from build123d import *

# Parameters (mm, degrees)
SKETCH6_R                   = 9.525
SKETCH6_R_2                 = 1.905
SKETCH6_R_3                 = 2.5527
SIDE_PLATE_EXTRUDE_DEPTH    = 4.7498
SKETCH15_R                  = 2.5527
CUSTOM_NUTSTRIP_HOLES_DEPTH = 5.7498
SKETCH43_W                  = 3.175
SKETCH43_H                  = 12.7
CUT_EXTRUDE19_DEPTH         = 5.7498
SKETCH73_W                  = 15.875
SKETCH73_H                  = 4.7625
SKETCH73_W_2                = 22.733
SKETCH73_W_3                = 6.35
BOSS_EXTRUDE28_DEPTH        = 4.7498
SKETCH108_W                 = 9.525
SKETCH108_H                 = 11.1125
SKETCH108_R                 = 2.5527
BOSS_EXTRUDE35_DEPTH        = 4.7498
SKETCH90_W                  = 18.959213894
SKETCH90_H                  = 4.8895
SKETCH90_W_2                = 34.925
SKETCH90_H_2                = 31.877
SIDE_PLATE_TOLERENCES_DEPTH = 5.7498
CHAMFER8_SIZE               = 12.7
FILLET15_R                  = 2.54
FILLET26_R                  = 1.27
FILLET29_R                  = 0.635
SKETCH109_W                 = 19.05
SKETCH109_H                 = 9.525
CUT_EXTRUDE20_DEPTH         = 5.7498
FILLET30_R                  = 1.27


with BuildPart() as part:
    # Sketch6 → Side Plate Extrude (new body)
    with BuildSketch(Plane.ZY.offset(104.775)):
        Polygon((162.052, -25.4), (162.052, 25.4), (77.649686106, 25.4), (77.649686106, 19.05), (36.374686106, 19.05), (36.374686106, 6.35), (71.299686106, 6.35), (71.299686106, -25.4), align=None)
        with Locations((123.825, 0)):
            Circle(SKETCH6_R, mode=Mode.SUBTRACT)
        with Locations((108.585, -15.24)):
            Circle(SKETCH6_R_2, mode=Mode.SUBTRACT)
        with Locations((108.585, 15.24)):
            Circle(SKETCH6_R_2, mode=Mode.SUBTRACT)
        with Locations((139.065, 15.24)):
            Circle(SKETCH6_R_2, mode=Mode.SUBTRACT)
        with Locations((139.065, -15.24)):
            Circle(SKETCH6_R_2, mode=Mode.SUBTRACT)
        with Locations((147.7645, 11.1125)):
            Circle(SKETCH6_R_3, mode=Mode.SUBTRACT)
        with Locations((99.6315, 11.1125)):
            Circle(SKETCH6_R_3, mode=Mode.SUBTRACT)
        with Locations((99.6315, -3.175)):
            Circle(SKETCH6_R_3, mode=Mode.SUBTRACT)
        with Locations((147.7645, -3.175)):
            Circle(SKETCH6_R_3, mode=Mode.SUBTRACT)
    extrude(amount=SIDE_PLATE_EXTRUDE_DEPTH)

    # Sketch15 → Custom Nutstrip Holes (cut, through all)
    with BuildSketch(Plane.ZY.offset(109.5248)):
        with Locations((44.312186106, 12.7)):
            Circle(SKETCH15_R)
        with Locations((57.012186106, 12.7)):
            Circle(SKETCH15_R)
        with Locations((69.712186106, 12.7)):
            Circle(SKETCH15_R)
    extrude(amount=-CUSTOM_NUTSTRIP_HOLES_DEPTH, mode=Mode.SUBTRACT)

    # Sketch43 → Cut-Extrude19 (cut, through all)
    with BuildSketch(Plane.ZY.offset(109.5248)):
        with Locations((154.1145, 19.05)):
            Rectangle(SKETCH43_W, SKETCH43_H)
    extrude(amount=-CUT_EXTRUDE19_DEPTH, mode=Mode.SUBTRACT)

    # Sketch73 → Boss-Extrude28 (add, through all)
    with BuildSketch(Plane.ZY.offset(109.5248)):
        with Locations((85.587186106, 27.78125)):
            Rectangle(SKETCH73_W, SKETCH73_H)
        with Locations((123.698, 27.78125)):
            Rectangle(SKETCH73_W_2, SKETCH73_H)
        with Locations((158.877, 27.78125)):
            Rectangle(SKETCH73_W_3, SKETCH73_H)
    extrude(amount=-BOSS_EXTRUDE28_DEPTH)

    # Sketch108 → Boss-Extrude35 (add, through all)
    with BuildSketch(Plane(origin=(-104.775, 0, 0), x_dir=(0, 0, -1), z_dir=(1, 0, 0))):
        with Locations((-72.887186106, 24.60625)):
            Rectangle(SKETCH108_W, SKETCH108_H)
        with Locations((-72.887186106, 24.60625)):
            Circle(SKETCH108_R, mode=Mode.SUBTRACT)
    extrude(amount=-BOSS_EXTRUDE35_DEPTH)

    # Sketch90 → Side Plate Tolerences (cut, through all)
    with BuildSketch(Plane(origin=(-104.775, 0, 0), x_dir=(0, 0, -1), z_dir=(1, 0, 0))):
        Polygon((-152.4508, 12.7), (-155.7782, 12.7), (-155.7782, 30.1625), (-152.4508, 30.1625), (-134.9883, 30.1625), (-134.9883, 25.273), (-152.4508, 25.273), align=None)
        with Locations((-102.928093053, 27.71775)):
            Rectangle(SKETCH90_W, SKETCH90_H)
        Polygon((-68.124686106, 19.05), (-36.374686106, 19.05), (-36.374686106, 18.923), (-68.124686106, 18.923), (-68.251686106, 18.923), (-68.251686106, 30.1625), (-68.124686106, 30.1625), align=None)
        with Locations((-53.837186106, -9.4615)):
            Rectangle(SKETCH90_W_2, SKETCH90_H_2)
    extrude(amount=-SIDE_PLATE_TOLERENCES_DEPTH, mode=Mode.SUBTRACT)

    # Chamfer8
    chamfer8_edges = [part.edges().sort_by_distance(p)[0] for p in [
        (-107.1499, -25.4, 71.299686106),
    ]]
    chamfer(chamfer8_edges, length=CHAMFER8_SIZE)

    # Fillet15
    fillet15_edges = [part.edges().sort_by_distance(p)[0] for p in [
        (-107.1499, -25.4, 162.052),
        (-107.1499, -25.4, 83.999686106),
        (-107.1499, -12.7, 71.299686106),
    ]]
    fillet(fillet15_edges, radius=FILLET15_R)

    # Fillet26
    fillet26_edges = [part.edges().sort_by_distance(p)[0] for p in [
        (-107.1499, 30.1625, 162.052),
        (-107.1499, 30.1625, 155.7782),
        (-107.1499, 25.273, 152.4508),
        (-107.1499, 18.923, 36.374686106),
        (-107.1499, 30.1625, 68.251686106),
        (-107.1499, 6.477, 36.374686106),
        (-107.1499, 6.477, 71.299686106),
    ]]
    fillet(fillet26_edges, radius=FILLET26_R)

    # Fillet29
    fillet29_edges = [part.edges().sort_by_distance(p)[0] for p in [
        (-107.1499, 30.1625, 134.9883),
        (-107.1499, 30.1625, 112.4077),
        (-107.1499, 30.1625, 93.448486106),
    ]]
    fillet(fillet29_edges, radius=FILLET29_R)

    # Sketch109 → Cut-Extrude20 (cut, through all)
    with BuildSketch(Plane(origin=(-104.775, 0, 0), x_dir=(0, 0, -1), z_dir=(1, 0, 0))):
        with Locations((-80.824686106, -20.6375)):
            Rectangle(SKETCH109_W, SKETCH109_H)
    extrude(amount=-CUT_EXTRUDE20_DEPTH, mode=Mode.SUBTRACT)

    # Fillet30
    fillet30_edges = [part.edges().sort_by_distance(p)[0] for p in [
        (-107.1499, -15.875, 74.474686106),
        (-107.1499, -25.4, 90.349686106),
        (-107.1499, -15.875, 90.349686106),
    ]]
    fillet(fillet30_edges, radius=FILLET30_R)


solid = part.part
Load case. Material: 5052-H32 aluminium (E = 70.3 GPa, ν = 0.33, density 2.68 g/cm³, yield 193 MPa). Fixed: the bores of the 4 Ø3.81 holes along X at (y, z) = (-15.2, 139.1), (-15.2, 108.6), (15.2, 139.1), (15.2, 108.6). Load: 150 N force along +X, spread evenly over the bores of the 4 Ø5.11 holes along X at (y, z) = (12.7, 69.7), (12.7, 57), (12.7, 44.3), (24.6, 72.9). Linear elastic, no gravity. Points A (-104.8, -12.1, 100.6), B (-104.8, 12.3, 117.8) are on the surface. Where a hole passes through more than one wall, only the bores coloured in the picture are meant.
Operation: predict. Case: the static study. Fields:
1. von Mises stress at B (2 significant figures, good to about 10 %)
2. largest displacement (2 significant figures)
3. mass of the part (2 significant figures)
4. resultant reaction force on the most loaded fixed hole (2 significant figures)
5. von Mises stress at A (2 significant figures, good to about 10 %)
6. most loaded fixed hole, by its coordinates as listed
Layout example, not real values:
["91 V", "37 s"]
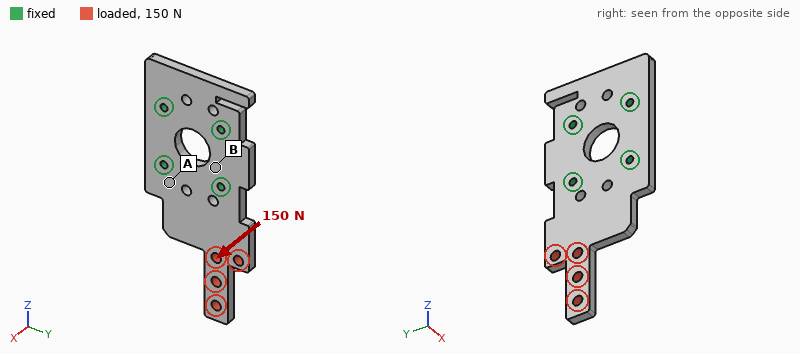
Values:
["8.0 MPa", "0.52 mm", "58 g", "180 N", "29 MPa", "(15.2, 108.6)"]
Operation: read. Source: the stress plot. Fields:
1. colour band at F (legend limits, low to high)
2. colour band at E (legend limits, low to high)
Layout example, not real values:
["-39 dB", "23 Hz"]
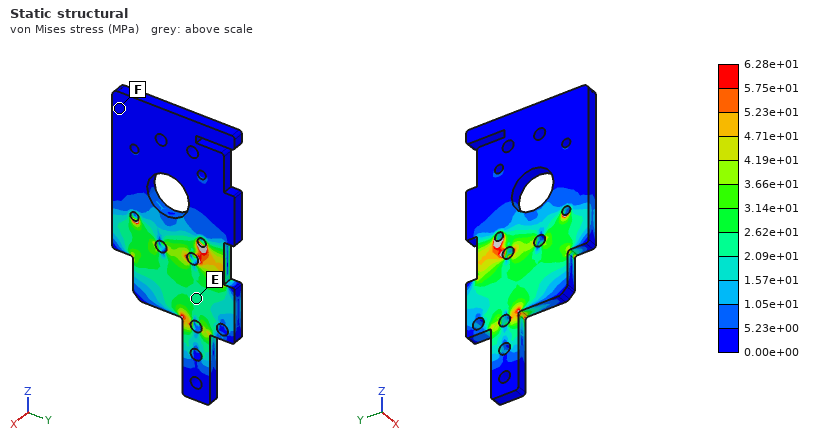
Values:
["0.00e+00 to 5.23e+00 MPa", "2.09e+01 to 2.62e+01 MPa"]
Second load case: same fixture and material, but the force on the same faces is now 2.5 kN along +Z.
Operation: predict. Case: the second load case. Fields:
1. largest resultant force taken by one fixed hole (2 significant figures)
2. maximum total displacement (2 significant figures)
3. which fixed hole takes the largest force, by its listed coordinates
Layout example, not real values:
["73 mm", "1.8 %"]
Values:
["2.0 kN", "34 µm", "(15.2, 108.6)"]
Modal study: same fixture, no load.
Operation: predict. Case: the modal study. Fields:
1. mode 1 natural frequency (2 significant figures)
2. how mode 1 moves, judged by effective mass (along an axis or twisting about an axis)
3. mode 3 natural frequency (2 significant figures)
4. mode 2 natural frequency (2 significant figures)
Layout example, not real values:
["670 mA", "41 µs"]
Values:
["1200 Hz", "along X", "5100 Hz", "3900 Hz"]
